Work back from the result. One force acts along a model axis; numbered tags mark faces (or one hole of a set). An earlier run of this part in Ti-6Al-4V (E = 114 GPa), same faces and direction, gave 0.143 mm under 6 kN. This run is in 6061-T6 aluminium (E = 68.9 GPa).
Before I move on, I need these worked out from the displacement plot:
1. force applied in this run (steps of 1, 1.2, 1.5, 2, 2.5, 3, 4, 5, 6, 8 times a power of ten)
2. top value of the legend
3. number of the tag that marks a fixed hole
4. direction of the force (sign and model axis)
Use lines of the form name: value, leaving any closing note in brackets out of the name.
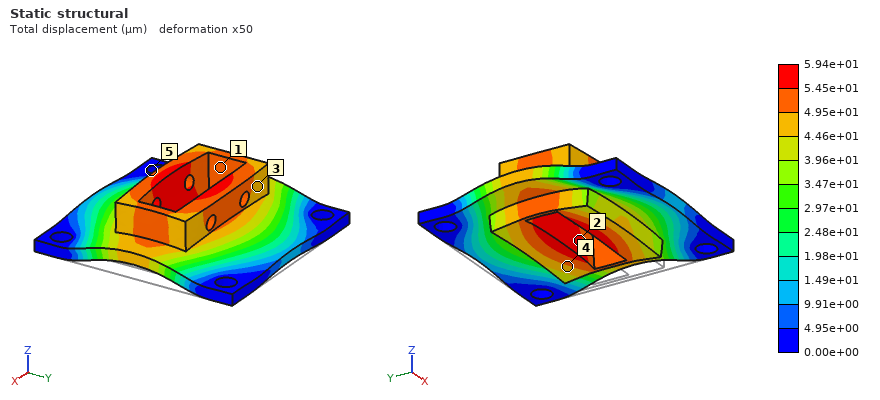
force applied in this run: 1.5 kN
top value of the legend: 5.94e+01 µm
number of the tag that marks a fixed hole: 5
direction of the force: +Z
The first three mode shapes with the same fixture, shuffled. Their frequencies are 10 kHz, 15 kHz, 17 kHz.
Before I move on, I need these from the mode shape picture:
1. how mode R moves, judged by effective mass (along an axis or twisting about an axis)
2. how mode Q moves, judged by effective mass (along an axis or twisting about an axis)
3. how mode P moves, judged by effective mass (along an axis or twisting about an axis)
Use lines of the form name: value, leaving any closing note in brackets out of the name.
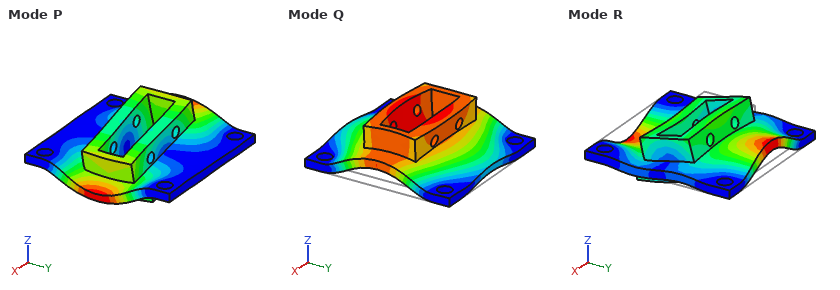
how mode R moves, judged by effective mass: twisting about X
how mode Q moves, judged by effective mass: along Z
how mode P moves, judged by effective mass: twisting about Y
